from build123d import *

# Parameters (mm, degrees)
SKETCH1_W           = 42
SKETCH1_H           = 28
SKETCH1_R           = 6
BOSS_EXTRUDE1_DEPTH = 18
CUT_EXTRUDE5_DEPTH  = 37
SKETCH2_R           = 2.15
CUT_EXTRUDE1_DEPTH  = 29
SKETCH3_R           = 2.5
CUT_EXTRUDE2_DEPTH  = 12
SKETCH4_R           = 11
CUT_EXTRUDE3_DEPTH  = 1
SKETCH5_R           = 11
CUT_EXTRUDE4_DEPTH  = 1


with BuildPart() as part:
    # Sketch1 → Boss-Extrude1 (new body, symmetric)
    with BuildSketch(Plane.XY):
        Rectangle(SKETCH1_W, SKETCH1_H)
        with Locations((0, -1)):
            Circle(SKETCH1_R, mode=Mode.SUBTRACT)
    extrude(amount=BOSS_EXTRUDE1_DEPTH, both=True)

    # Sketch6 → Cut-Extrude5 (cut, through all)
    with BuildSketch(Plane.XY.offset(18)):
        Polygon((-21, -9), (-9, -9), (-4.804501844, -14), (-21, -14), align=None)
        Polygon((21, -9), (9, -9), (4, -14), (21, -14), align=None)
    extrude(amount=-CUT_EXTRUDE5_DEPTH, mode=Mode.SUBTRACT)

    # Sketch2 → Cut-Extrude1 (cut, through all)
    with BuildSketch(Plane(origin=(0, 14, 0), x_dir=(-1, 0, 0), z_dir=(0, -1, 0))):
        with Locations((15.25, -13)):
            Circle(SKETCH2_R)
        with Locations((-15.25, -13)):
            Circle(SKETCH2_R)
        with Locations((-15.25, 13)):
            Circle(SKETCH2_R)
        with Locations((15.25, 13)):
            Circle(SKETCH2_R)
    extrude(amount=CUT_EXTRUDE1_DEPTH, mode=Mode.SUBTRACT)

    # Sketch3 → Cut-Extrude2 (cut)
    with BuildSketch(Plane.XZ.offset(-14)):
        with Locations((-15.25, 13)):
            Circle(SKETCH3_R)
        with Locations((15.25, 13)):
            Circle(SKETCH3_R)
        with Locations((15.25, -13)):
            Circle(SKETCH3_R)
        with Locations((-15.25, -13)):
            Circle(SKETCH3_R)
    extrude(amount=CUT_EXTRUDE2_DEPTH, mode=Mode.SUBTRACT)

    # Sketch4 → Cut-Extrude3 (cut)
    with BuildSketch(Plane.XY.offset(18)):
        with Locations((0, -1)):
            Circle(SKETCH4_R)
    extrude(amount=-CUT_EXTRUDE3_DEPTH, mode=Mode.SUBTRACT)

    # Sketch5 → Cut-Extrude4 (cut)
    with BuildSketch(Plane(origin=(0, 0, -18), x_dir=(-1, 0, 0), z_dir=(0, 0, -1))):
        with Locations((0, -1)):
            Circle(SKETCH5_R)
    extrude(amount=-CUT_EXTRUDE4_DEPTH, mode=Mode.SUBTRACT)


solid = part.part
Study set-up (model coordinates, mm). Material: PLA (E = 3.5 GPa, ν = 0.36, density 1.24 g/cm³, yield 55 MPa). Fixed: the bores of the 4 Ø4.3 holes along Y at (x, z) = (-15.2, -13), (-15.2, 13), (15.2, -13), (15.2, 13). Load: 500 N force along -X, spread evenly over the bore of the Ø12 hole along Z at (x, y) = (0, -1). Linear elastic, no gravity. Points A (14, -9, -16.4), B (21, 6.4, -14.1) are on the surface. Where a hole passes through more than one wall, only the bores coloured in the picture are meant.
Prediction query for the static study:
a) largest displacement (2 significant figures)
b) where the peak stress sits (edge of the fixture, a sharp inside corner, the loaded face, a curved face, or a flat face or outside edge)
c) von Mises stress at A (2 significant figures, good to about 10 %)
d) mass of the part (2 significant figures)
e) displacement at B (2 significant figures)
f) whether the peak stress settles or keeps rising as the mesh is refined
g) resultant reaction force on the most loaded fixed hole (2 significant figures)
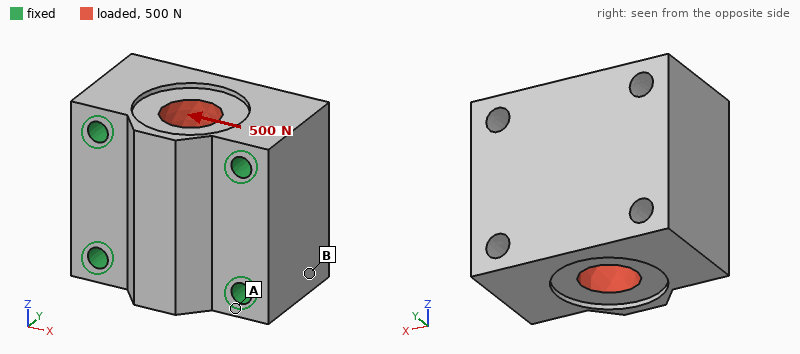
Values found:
3.8 µm
edge of the fixture
0.42 MPa
38 g
2.0 µm
keeps rising
130 N
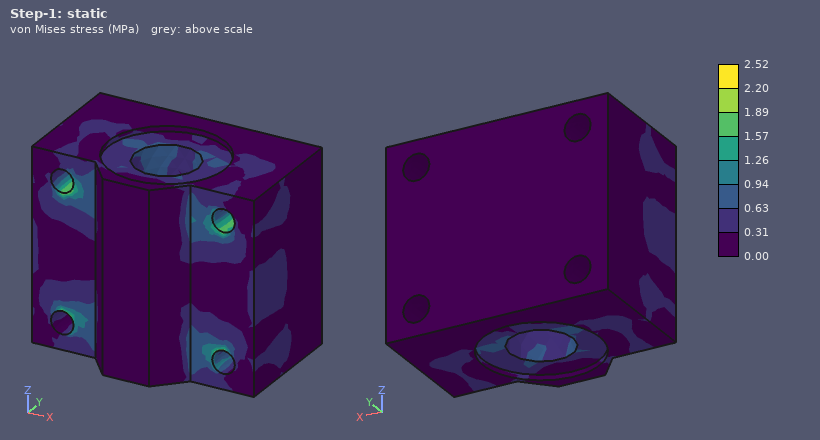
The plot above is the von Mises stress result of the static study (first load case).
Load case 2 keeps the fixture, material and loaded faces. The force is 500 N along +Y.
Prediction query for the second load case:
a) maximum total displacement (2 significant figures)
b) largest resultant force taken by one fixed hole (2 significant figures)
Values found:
6.3 µm
130 N
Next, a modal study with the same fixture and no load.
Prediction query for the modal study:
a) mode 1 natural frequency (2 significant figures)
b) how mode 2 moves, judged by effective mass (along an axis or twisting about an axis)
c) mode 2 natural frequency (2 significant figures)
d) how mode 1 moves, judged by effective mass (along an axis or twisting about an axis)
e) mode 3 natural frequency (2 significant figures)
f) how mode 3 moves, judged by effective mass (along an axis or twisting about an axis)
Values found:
9400 Hz
along Z
9900 Hz
along X
11 kHz
along Y
